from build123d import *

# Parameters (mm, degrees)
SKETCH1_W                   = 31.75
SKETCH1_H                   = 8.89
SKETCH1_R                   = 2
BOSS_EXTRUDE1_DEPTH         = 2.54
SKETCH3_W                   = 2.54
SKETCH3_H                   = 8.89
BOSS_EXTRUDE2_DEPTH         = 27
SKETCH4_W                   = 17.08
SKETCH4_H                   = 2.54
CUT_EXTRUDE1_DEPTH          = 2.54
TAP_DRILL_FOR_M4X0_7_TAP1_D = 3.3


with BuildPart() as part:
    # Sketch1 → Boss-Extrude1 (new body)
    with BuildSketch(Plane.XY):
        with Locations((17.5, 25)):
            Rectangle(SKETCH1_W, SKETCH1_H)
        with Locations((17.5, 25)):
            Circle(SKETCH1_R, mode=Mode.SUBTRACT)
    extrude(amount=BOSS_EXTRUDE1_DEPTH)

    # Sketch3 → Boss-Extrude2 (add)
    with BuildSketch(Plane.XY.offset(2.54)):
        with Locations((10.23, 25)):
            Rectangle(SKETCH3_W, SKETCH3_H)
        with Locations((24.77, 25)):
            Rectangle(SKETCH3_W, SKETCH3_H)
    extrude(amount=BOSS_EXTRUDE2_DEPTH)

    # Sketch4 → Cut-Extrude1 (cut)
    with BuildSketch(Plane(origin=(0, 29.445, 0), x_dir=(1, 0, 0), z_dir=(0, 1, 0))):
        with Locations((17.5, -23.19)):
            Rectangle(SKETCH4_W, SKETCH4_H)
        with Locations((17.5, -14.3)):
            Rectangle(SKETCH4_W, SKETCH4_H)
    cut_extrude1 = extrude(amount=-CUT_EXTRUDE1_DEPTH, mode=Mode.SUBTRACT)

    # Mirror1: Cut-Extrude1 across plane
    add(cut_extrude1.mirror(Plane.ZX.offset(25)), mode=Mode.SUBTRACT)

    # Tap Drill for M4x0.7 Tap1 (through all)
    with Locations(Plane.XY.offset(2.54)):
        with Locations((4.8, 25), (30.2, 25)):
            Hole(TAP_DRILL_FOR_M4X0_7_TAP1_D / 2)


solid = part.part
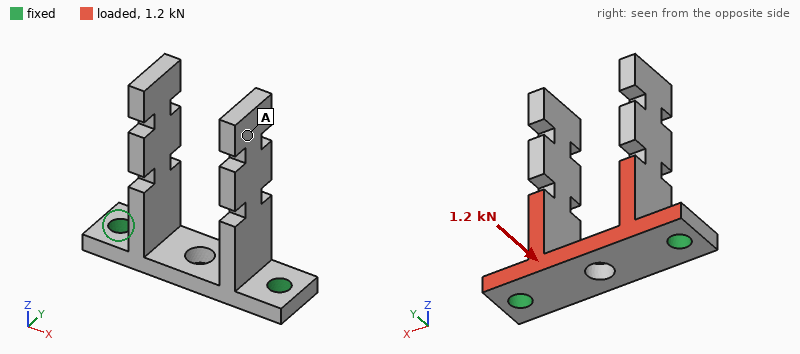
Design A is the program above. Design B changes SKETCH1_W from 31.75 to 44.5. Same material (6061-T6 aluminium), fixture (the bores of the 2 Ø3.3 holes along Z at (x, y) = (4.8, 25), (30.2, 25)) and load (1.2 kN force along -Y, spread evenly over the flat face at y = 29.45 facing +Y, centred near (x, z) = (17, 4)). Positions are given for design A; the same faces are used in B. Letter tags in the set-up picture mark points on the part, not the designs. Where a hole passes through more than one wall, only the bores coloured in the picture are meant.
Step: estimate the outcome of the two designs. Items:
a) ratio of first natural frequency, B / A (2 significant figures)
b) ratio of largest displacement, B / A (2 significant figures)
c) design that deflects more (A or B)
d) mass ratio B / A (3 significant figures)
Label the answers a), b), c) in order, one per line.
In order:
a) 1.00
b) 0.79
c) A
d) 1.17
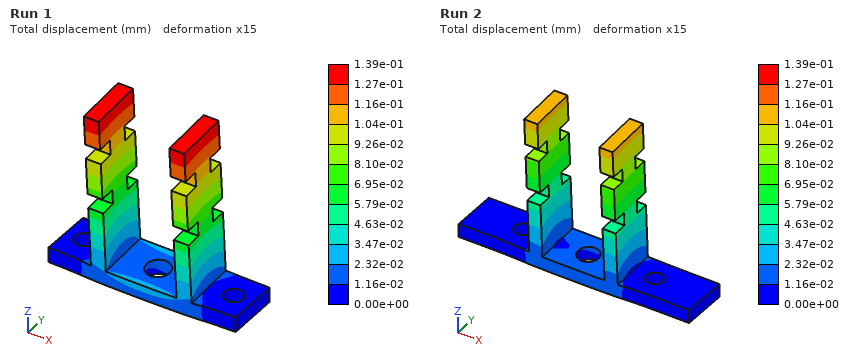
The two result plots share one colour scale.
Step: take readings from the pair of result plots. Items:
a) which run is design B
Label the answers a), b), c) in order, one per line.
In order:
a) Run 2
